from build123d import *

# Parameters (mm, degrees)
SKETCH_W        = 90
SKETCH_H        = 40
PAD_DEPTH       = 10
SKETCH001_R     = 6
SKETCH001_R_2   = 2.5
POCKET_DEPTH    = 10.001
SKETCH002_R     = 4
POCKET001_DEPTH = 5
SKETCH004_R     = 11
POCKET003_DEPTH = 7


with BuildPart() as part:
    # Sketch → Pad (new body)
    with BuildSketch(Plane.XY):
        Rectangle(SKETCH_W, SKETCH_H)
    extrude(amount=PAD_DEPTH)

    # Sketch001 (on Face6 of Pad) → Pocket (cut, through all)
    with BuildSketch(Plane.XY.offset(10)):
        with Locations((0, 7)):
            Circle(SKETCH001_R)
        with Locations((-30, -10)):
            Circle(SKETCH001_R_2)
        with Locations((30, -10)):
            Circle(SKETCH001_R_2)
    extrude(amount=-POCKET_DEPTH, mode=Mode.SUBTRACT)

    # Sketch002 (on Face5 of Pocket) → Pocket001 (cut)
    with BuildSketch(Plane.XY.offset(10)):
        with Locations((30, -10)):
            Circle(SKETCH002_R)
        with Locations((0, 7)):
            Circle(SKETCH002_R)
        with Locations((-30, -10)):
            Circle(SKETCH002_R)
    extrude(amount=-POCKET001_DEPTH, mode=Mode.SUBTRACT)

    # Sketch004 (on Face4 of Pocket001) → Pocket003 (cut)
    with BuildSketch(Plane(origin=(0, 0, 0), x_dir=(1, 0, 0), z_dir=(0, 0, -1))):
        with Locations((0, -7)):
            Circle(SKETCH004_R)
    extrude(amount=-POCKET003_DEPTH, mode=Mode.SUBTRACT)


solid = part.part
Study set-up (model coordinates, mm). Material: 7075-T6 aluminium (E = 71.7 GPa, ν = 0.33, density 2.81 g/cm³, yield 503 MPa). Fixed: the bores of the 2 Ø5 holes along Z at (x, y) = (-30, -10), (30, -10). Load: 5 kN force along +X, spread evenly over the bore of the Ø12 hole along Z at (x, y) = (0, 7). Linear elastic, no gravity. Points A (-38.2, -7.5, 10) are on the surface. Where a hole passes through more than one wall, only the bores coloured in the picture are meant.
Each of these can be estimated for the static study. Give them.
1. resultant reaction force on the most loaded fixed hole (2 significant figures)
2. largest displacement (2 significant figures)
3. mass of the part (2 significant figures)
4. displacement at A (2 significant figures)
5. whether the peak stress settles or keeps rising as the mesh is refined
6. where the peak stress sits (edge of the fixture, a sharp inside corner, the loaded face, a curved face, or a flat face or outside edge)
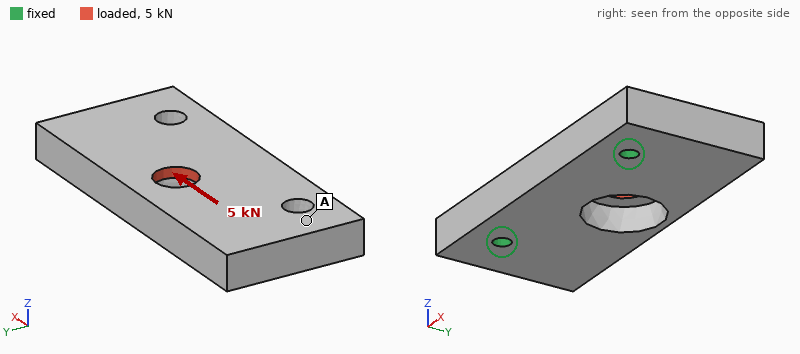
2.9 kN
20 µm
91 g
5.6 µm
keeps rising
edge of the fixture
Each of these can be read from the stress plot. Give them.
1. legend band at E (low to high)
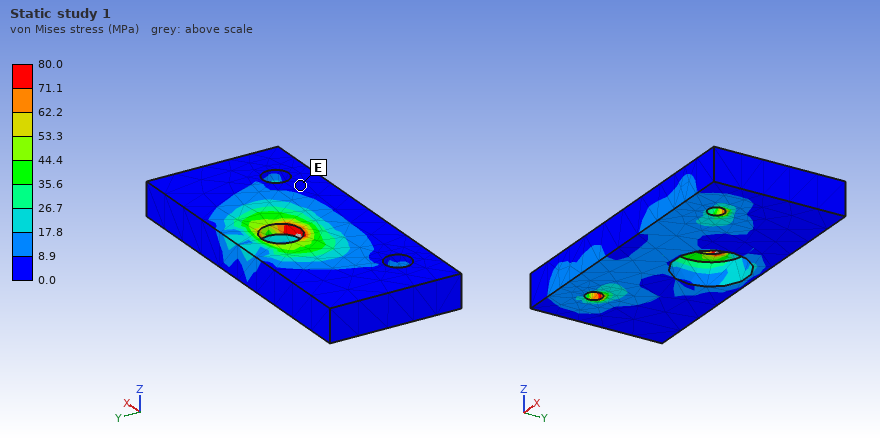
0.0 to 8.9 MPa
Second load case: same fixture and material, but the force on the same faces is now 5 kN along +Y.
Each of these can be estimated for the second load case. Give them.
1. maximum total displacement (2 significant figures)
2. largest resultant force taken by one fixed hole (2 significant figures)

95 µm
2.6 kN
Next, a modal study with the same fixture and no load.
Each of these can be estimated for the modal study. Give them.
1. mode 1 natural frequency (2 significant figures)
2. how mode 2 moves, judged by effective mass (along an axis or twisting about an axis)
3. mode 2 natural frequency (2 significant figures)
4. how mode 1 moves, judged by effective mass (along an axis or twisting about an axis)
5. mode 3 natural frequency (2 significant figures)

3900 Hz
twisting about Y
6400 Hz
along Z
8100 Hz
